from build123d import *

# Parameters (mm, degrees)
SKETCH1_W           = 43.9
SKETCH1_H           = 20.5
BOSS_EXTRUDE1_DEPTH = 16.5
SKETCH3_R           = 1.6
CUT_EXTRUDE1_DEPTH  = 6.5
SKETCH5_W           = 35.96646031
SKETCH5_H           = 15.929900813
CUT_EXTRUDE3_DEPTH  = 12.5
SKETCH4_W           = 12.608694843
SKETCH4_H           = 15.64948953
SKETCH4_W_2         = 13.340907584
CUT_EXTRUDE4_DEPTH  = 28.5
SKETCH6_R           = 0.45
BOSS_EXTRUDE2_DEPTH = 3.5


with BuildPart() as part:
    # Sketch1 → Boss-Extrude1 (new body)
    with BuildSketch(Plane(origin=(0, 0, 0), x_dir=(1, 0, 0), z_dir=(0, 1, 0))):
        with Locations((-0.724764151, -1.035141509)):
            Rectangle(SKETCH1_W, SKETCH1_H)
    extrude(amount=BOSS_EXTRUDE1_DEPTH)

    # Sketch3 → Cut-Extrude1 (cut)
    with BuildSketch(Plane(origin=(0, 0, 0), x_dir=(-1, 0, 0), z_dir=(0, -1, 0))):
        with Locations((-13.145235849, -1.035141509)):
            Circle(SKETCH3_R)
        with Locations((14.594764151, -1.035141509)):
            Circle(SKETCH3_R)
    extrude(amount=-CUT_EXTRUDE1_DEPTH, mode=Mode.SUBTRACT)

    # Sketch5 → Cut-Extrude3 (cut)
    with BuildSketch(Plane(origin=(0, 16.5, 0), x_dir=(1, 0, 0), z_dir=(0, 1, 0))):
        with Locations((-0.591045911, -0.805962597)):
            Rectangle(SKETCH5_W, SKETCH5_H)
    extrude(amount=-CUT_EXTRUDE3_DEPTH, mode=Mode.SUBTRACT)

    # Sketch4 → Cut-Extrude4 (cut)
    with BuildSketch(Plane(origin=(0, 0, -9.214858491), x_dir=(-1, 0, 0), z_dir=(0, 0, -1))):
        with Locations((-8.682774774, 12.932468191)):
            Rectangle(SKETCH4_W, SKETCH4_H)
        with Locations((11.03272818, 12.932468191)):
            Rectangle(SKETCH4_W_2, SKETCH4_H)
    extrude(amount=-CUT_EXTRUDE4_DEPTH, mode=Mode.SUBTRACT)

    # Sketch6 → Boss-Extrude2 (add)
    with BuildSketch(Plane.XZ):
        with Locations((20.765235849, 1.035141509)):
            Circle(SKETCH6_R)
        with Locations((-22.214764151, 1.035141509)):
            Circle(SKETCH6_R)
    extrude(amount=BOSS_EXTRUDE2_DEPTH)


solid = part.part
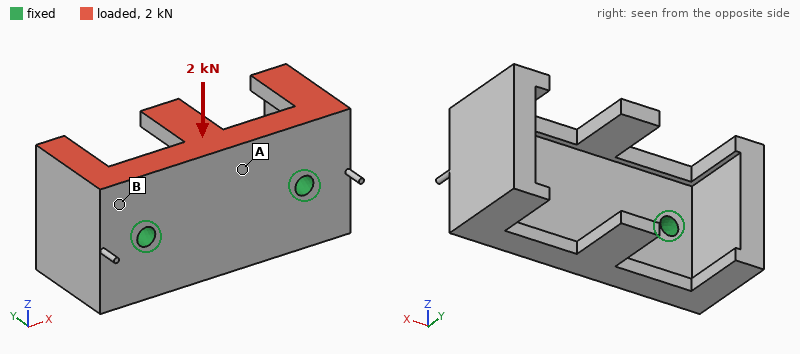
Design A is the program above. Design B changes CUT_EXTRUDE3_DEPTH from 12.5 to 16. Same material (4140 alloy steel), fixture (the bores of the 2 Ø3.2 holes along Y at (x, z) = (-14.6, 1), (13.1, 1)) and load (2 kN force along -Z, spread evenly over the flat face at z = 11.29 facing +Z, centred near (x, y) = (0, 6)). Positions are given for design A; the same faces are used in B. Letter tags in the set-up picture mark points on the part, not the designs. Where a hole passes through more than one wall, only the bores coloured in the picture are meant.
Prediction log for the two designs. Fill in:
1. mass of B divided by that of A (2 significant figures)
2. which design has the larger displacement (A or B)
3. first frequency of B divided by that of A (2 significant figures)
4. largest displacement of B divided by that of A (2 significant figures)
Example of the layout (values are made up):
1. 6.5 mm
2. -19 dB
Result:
1. 0.69
2. B
3. 0.089
4. 31
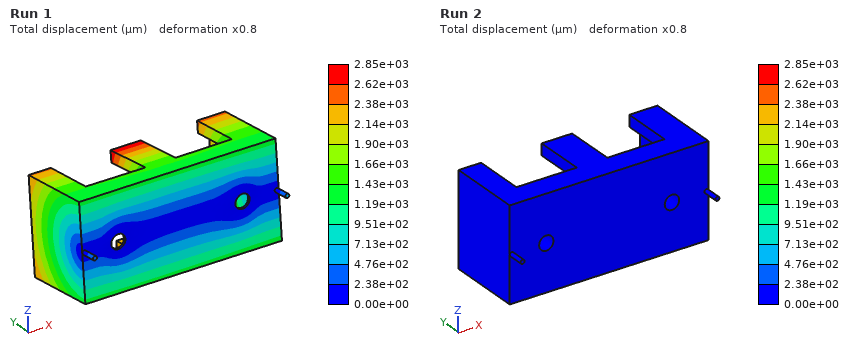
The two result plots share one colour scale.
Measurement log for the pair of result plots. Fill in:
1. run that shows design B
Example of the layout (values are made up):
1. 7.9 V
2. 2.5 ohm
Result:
1. Run 1
